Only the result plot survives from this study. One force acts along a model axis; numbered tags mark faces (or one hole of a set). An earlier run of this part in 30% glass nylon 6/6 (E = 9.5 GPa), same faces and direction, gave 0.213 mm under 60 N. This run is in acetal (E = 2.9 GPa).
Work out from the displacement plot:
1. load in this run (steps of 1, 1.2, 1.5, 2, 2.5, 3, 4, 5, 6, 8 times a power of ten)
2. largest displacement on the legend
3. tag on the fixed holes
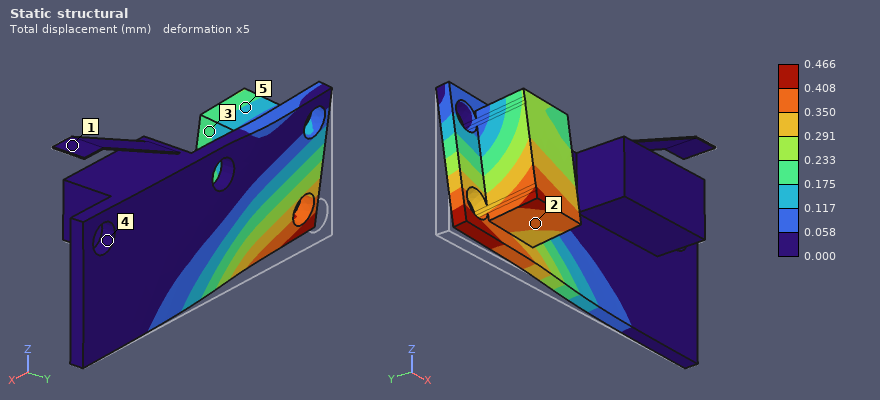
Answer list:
40 N
0.466 mm
4
